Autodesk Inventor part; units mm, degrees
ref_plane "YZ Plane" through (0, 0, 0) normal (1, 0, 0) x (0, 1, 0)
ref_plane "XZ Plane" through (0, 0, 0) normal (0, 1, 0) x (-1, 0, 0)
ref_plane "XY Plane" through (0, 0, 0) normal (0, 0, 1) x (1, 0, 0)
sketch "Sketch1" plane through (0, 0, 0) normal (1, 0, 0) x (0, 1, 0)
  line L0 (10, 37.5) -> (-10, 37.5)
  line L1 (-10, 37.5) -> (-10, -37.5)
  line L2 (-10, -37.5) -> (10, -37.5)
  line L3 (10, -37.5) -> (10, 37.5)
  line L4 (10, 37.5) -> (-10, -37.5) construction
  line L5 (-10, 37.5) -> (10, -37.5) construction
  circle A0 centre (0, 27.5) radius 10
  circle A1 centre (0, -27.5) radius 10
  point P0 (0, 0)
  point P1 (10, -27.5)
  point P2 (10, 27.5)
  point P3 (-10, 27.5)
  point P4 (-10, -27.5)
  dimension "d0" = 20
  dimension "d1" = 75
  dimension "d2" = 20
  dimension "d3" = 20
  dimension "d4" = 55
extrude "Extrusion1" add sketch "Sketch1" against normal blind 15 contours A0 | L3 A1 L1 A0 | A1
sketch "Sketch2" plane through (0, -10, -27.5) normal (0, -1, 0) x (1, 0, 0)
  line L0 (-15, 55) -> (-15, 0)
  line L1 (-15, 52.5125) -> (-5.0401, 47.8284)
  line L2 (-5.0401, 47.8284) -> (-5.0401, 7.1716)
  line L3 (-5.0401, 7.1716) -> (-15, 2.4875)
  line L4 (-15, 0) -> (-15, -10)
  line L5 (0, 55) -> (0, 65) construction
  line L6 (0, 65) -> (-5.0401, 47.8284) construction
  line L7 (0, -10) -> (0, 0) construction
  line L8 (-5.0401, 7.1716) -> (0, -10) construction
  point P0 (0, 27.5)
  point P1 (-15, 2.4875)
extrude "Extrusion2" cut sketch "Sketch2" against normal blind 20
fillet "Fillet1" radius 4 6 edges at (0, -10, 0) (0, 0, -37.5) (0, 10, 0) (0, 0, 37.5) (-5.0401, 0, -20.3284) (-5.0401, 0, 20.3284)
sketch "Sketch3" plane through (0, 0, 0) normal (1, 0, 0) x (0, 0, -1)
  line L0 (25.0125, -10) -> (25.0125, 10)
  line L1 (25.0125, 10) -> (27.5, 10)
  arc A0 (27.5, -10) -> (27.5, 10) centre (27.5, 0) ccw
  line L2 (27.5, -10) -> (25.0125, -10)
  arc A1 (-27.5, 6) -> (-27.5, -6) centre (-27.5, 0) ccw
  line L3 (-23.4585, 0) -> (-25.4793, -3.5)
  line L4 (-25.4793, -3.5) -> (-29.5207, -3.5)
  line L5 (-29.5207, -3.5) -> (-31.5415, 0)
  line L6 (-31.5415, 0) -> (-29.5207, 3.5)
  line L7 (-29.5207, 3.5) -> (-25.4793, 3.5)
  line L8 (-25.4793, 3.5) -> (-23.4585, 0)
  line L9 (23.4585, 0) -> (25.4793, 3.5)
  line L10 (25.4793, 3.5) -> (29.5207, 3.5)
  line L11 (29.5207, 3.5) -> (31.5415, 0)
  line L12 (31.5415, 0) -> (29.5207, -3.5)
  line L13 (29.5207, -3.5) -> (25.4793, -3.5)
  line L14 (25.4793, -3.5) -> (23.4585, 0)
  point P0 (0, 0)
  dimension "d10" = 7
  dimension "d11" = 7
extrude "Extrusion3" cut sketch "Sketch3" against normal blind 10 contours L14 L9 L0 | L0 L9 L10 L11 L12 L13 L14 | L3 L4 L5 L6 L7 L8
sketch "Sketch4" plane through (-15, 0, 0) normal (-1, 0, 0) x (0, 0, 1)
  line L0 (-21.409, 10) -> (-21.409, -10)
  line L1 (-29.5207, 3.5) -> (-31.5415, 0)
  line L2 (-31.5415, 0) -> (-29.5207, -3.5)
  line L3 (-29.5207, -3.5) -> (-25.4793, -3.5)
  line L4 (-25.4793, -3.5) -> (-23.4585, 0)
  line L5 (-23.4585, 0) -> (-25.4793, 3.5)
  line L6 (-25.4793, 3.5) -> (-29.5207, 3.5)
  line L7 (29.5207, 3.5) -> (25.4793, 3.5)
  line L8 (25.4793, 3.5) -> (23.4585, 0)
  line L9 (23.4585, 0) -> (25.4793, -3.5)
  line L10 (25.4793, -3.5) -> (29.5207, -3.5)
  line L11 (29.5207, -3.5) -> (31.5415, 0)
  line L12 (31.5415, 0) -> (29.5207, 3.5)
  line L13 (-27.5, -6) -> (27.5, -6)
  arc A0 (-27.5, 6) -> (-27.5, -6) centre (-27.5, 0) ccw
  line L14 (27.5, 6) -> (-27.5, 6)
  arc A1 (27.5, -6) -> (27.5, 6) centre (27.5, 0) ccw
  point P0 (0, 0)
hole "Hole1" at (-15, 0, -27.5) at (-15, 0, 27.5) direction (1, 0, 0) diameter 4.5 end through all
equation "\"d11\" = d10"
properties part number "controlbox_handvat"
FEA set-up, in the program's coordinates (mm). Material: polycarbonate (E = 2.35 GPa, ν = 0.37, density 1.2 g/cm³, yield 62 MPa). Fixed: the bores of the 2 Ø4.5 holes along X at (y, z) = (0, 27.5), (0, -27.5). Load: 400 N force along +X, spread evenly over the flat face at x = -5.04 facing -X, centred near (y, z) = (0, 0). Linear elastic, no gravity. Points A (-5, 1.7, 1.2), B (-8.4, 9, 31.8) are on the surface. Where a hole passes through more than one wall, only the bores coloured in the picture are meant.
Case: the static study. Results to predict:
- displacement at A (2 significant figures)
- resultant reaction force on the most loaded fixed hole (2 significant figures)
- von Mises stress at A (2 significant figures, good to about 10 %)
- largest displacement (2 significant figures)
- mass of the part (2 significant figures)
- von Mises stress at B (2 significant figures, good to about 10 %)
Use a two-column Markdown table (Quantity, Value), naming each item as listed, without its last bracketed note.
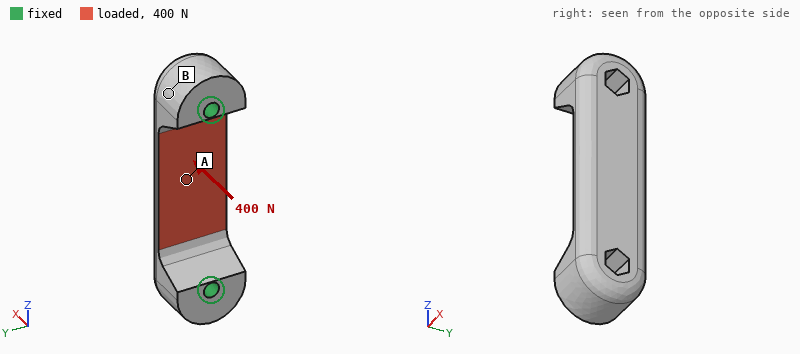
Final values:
| Quantity | Value |
|---|---|
| displacement at A | 0.34 mm |
| resultant reaction force on the most loaded fixed hole | 300 N |
| von Mises stress at A | 9.0 MPa |
| largest displacement | 0.38 mm |
| mass of the part | 13 g |
| von Mises stress at B | 2.0 MPa |
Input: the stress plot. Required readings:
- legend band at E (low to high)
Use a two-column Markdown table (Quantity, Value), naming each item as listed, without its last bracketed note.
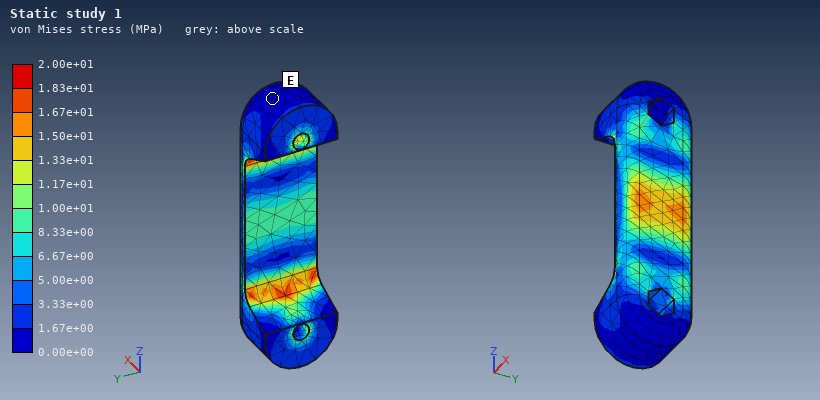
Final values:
| Quantity | Value |
|---|---|
| legend band at E | 0.00e+00 to 1.67e+00 MPa |
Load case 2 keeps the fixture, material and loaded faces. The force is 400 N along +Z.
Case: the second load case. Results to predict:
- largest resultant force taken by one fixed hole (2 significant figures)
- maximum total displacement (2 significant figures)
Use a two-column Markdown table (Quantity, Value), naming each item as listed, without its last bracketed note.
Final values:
| Quantity | Value |
|---|---|
| largest resultant force taken by one fixed hole | 200 N |
| maximum total displacement | 0.12 mm |
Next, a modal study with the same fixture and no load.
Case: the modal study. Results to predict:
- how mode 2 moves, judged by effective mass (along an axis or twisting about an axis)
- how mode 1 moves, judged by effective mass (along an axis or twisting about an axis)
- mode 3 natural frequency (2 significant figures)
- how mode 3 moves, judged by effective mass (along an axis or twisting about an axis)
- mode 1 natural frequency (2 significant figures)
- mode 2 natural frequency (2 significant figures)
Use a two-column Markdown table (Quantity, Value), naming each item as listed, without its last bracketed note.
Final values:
| Quantity | Value |
|---|---|
| how mode 2 moves, judged by effective mass | along X |
| how mode 1 moves, judged by effective mass | along Y |
| mode 3 natural frequency | 3400 Hz |
| how mode 3 moves, judged by effective mass | along Z |
| mode 1 natural frequency | 2700 Hz |
| mode 2 natural frequency | 3000 Hz |
